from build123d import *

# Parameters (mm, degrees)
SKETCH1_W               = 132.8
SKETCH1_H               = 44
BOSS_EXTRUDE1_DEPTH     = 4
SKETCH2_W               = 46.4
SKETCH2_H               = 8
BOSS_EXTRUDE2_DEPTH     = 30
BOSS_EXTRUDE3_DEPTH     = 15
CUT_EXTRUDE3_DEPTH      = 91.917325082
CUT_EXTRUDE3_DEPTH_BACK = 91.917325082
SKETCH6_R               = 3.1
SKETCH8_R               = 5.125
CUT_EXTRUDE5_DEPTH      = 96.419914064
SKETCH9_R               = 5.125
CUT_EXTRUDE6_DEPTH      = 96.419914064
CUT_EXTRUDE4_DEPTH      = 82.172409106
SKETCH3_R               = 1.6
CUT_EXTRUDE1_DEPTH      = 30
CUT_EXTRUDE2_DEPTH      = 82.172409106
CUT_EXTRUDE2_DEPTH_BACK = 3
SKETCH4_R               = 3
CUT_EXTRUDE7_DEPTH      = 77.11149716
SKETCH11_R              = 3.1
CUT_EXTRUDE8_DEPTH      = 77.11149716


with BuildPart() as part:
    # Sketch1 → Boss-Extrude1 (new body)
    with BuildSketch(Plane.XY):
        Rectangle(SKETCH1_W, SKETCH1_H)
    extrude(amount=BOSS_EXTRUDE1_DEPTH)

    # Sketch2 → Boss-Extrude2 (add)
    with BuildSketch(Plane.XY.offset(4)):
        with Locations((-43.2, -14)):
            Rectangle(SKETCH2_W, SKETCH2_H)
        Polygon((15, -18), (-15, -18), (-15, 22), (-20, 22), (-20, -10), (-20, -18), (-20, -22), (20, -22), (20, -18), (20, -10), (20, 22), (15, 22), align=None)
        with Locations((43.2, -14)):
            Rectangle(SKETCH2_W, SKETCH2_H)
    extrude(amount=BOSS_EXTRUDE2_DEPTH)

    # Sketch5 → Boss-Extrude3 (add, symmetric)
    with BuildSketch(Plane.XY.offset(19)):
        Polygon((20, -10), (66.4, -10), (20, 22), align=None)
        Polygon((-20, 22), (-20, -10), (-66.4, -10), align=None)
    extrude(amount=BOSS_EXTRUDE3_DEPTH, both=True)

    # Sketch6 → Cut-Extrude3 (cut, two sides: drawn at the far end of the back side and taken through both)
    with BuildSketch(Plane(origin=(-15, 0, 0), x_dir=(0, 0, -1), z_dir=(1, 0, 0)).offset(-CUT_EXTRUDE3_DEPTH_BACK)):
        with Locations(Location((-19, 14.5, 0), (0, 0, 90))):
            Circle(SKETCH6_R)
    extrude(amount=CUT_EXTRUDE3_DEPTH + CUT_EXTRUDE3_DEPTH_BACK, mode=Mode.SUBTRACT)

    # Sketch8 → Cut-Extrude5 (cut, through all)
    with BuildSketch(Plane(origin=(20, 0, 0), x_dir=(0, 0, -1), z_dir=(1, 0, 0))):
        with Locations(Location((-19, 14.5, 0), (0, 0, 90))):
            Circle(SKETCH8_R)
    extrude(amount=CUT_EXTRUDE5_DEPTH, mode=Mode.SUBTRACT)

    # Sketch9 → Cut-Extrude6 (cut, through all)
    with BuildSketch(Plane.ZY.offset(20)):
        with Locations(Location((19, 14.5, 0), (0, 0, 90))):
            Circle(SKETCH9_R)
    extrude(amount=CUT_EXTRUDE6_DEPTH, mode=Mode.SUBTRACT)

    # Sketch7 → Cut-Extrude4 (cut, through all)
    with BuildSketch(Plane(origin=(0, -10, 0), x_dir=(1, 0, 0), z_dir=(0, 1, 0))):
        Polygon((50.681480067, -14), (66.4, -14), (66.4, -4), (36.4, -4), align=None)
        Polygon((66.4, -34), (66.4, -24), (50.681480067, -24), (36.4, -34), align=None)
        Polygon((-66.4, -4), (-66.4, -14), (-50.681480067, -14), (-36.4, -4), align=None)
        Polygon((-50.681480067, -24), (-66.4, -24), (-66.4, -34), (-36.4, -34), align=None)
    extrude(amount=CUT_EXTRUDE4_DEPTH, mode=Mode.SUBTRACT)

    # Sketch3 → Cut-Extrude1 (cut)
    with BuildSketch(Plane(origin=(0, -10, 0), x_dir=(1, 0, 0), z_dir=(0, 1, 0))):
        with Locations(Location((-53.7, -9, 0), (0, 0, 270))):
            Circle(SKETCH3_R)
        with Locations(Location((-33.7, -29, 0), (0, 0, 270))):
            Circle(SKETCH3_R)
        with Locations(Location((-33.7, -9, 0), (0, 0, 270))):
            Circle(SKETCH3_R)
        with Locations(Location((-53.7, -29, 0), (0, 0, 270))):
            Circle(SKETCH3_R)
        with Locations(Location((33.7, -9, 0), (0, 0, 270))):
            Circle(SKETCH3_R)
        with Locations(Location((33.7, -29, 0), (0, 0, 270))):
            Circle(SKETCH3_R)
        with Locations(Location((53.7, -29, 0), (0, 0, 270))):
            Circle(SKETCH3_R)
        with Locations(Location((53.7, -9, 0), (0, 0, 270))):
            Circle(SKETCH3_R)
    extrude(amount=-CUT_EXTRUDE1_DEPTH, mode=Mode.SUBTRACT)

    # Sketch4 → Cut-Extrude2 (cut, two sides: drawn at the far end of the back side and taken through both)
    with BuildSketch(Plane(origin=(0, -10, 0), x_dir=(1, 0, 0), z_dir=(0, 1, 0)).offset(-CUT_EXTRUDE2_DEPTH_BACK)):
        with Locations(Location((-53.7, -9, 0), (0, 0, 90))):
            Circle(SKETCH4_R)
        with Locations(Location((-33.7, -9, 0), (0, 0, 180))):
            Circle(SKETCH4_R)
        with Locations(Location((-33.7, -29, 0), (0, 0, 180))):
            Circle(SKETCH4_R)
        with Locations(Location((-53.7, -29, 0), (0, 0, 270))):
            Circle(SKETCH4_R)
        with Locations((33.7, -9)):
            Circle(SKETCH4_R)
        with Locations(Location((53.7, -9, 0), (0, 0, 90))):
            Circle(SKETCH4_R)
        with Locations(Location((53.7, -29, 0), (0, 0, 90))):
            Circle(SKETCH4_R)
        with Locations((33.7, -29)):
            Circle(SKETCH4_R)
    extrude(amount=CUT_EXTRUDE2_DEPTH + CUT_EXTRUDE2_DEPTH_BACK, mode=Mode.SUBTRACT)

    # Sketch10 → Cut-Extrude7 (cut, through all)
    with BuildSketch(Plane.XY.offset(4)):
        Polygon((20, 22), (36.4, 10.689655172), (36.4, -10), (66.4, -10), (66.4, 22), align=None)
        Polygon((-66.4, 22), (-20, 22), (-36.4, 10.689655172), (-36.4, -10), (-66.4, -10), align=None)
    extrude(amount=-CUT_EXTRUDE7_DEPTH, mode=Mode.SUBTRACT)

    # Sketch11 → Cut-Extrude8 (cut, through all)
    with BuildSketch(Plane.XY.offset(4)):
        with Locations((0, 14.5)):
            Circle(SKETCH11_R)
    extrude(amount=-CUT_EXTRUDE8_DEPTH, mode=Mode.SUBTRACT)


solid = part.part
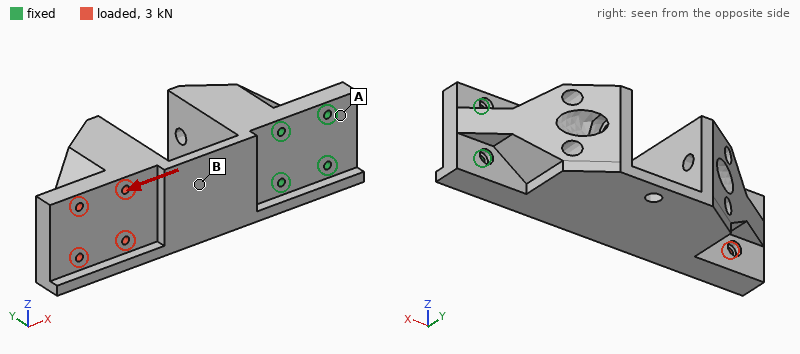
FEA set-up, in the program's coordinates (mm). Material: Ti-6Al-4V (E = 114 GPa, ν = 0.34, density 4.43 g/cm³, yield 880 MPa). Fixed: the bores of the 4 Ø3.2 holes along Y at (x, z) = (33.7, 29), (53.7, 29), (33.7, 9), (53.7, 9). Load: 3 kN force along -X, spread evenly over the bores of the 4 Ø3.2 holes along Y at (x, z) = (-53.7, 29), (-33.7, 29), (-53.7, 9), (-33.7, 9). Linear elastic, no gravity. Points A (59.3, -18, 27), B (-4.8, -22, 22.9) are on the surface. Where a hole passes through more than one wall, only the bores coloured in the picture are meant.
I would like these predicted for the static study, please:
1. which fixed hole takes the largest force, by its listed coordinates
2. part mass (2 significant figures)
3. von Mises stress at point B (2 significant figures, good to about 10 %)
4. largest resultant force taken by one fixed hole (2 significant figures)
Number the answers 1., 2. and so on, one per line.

1. (33.7, 29)
2. 380 g
3. 16 MPa
4. 1.3 kN
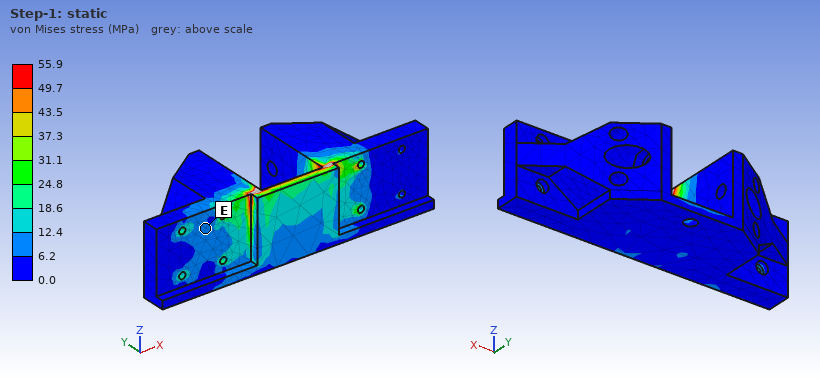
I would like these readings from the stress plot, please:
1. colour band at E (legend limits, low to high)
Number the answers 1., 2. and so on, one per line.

1. 6.2 to 12.4 MPa
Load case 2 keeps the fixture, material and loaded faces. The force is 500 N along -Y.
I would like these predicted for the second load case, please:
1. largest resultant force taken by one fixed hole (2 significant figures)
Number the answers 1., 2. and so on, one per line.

1. 1.2 kN
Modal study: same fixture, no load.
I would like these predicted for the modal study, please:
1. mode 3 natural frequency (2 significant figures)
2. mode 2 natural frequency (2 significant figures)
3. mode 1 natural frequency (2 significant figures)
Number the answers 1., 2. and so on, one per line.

1. 2800 Hz
2. 1300 Hz
3. 1100 Hz
